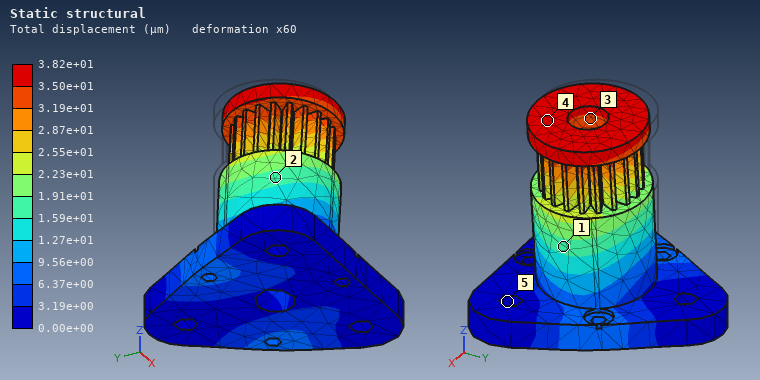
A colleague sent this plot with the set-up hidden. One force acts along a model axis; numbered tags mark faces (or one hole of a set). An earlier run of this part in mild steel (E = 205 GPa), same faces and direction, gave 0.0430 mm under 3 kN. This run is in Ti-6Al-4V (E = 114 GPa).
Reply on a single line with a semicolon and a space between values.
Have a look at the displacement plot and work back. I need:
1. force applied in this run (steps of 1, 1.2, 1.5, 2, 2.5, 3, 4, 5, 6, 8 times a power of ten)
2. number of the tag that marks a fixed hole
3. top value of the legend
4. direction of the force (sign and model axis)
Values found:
1.5 kN; 5; 3.82e+01 µm; +X
